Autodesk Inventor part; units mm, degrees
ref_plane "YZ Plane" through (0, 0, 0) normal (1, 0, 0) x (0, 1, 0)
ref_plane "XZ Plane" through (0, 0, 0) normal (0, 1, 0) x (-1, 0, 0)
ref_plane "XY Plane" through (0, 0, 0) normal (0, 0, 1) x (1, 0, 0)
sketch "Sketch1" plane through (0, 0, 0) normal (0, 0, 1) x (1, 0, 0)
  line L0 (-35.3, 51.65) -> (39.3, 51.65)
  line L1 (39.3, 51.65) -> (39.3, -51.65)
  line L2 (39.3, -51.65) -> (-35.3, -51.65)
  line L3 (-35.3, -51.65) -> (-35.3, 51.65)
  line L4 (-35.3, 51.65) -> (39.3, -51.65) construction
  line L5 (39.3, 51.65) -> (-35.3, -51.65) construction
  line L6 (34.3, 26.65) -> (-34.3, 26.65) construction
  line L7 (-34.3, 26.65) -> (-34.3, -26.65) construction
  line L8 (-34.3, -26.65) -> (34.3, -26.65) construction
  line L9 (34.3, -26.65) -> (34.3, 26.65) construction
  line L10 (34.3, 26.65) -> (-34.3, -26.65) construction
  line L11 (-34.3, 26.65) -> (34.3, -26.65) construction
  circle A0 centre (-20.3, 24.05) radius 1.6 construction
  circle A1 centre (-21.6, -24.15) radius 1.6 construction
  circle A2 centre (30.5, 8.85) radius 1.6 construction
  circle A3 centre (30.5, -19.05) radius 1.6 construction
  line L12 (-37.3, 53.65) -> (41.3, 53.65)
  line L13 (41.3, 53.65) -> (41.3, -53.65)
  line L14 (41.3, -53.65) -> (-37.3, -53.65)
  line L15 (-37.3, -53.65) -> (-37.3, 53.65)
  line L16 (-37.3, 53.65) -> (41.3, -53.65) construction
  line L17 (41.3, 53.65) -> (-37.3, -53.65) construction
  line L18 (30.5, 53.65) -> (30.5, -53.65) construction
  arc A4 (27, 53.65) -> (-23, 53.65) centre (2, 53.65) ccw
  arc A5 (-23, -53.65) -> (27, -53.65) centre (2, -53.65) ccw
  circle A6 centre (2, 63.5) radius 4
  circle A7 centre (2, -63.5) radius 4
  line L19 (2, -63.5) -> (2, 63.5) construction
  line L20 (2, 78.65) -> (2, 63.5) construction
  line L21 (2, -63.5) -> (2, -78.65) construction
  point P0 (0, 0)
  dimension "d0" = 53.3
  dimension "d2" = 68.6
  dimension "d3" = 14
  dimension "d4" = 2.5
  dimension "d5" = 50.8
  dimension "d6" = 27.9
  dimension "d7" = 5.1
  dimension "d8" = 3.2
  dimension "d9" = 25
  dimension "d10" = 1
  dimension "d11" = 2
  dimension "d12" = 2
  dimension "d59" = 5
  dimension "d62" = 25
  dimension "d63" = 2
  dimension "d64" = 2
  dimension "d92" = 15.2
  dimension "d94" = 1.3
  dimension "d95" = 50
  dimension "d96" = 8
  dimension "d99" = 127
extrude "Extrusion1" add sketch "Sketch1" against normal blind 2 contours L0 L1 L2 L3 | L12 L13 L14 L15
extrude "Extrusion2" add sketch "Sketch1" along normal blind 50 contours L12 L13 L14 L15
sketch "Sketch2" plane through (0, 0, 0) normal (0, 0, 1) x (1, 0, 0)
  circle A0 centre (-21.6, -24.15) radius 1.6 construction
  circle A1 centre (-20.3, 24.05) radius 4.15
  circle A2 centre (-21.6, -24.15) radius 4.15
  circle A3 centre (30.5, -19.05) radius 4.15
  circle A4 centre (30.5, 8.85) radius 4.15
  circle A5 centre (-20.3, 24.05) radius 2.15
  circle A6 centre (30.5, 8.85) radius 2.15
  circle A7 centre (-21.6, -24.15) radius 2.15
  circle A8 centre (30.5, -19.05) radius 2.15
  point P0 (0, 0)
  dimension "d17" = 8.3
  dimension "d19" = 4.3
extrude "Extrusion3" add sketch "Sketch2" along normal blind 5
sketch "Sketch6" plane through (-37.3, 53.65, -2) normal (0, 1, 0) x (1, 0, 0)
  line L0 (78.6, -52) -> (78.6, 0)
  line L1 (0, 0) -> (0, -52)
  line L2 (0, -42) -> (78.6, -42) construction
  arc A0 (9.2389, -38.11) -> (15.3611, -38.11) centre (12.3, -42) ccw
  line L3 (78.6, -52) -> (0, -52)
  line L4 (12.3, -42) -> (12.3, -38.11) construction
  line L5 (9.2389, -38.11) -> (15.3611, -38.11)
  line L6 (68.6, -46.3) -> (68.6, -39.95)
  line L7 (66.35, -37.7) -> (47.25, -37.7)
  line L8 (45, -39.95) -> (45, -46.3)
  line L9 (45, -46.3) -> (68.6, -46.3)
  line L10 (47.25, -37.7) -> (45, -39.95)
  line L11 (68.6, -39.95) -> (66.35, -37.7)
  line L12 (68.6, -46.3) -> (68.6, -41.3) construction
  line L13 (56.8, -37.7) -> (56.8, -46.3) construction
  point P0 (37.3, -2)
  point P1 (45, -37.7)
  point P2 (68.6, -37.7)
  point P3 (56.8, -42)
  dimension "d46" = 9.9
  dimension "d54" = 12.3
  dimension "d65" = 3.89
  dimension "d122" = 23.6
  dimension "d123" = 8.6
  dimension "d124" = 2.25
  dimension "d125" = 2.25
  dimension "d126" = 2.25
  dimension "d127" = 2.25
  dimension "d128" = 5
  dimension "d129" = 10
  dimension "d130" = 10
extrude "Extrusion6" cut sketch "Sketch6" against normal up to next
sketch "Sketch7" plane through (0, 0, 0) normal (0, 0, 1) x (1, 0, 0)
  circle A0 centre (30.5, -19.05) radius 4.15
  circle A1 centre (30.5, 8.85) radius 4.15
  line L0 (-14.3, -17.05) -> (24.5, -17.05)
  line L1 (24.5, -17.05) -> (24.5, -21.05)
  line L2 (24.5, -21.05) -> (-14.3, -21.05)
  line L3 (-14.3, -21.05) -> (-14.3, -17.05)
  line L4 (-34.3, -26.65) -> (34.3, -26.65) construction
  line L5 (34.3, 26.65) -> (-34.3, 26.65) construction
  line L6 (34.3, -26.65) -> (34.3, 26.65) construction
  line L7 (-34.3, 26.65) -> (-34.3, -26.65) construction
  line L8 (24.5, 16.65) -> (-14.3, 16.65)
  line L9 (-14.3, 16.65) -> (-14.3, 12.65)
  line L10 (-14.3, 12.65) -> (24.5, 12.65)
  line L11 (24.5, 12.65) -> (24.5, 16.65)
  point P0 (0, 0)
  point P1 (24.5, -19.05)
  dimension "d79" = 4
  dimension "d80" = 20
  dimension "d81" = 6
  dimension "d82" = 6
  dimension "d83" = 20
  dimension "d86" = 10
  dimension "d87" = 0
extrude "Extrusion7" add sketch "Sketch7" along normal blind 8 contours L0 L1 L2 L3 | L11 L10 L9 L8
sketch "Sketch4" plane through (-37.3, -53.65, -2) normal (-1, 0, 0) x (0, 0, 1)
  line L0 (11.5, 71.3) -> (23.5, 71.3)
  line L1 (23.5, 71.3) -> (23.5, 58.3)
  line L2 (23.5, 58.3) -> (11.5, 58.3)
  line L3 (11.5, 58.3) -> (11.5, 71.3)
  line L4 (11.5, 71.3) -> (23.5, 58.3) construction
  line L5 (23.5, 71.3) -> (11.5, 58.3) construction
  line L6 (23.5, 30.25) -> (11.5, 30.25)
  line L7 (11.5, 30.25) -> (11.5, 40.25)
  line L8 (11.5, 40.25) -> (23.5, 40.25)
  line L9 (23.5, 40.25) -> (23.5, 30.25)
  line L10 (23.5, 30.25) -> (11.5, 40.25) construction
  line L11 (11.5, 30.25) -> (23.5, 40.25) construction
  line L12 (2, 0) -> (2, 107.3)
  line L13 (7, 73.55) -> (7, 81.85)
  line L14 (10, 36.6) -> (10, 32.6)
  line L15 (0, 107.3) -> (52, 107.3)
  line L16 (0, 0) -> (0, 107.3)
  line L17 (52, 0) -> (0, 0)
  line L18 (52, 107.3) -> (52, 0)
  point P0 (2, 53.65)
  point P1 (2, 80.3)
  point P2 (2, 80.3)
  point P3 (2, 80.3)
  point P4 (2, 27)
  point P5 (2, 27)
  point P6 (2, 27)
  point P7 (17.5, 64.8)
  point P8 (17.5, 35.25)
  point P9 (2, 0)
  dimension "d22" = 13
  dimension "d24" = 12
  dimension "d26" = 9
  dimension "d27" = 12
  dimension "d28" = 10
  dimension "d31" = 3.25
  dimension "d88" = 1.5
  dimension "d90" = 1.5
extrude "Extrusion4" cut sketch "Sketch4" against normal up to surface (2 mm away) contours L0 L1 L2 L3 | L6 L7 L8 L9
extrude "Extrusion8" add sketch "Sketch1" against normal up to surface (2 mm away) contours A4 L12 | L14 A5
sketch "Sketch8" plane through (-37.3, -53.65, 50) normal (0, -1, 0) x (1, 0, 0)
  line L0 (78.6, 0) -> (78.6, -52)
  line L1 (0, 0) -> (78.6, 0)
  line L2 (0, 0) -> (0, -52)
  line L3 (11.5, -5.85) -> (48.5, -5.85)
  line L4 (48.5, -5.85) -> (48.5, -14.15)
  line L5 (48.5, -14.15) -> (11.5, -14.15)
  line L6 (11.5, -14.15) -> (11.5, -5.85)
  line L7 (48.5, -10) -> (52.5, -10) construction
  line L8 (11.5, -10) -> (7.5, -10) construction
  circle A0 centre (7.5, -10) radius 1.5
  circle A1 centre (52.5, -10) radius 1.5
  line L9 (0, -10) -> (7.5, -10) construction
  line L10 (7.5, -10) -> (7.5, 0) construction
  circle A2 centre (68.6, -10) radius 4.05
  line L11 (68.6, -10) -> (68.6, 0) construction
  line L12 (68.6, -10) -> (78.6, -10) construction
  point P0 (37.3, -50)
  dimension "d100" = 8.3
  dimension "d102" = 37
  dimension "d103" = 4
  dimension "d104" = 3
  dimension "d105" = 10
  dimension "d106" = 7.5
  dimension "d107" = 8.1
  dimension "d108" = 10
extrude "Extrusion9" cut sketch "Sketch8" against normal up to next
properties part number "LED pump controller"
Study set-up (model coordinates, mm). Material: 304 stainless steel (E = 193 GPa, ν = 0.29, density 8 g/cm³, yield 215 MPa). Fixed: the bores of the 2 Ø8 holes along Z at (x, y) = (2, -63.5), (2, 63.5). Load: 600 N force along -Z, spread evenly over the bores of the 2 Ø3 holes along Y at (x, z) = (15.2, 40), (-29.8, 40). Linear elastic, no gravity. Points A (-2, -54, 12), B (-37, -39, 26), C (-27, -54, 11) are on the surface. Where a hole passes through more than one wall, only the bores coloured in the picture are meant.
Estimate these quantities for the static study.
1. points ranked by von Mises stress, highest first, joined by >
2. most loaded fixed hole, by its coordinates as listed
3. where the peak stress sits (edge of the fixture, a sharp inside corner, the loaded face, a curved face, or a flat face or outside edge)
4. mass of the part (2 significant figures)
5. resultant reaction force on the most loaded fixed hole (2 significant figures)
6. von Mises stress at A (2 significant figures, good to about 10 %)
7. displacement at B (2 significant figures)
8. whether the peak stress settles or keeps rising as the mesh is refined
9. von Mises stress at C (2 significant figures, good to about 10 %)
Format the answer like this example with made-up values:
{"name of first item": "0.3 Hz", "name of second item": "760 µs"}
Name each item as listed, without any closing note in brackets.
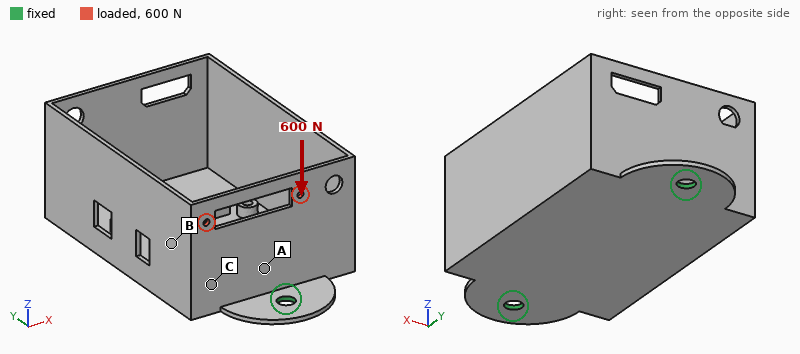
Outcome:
{"points ranked by von Mises stress, highest first, joined by >": "A > C > B", "most loaded fixed hole, by its coordinates as listed": "(2, -63.5)", "where the peak stress sits": "edge of the fixture", "mass of the part": "470 g", "resultant reaction force on the most loaded fixed hole": "580 N", "von Mises stress at A": "26 MPa", "displacement at B": "0.13 mm", "whether the peak stress settles or keeps rising as the mesh is refined": "keeps rising", "von Mises stress at C": "15 MPa"}
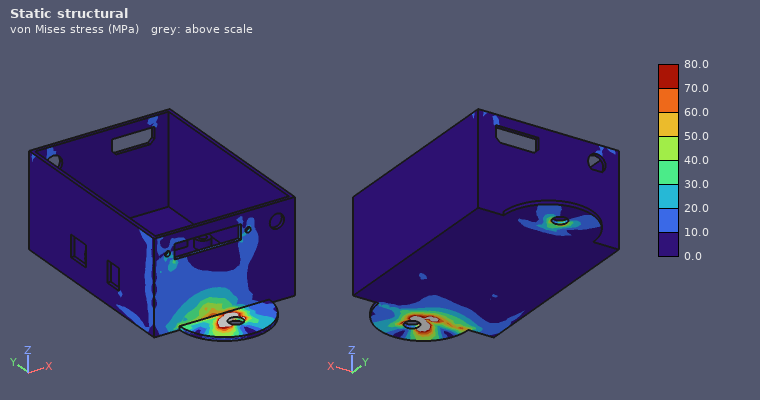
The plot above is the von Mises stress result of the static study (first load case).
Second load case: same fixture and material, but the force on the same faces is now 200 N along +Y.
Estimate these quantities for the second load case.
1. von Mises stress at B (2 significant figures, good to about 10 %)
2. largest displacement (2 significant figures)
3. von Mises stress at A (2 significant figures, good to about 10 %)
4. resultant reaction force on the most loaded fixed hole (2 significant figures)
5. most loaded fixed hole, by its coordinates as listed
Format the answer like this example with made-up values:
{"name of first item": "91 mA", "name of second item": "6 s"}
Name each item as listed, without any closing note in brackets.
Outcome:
{"von Mises stress at B": "9.8 MPa", "largest displacement": "0.11 mm", "von Mises stress at A": "17 MPa", "resultant reaction force on the most loaded fixed hole": "130 N", "most loaded fixed hole, by its coordinates as listed": "(2, -63.5)"}
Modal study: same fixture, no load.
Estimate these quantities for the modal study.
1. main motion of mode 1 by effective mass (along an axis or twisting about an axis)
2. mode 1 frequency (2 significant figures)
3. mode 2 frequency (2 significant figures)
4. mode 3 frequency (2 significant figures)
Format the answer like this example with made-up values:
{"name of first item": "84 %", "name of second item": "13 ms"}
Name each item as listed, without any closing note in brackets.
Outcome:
{"main motion of mode 1 by effective mass": "along X", "mode 1 frequency": "360 Hz", "mode 2 frequency": "680 Hz", "mode 3 frequency": "950 Hz"}
